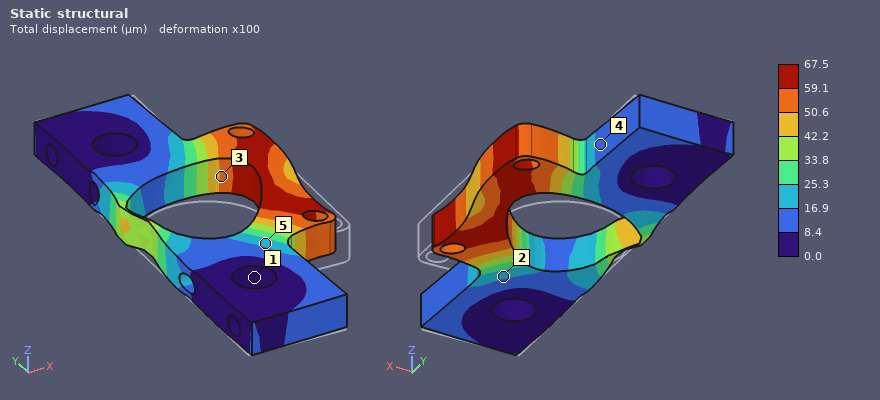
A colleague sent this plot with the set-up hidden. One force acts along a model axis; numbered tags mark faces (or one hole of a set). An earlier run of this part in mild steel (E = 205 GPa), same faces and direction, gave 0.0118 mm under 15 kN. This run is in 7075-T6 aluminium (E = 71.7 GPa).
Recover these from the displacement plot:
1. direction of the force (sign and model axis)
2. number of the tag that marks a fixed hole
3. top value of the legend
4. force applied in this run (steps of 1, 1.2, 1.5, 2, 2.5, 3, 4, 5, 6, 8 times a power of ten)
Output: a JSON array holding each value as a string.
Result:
["+Y", "1", "67.5 µm", "30 kN"]
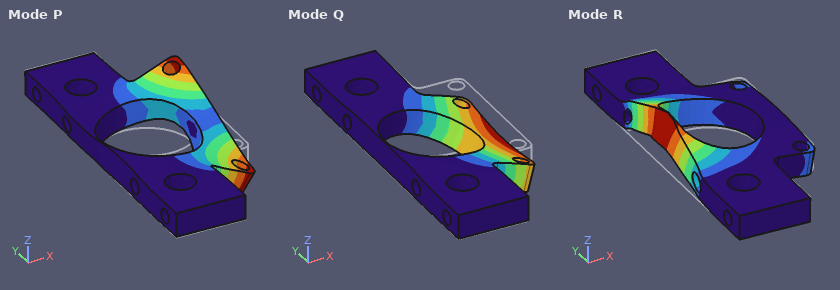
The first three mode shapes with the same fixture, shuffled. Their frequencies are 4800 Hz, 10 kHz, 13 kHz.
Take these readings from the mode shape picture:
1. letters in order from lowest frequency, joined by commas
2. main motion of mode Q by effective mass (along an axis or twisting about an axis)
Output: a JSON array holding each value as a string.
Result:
["Q, P, R", "along Z"]
